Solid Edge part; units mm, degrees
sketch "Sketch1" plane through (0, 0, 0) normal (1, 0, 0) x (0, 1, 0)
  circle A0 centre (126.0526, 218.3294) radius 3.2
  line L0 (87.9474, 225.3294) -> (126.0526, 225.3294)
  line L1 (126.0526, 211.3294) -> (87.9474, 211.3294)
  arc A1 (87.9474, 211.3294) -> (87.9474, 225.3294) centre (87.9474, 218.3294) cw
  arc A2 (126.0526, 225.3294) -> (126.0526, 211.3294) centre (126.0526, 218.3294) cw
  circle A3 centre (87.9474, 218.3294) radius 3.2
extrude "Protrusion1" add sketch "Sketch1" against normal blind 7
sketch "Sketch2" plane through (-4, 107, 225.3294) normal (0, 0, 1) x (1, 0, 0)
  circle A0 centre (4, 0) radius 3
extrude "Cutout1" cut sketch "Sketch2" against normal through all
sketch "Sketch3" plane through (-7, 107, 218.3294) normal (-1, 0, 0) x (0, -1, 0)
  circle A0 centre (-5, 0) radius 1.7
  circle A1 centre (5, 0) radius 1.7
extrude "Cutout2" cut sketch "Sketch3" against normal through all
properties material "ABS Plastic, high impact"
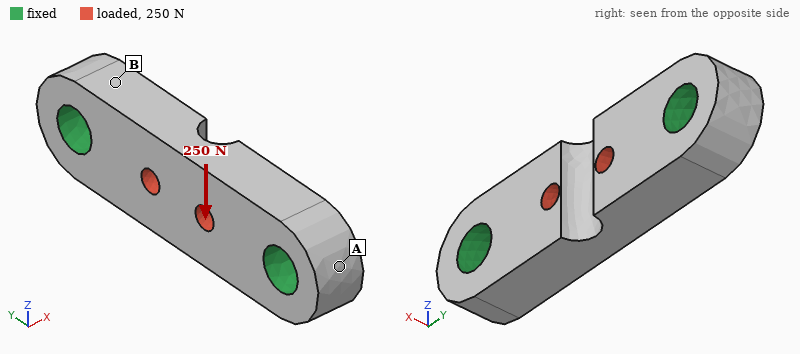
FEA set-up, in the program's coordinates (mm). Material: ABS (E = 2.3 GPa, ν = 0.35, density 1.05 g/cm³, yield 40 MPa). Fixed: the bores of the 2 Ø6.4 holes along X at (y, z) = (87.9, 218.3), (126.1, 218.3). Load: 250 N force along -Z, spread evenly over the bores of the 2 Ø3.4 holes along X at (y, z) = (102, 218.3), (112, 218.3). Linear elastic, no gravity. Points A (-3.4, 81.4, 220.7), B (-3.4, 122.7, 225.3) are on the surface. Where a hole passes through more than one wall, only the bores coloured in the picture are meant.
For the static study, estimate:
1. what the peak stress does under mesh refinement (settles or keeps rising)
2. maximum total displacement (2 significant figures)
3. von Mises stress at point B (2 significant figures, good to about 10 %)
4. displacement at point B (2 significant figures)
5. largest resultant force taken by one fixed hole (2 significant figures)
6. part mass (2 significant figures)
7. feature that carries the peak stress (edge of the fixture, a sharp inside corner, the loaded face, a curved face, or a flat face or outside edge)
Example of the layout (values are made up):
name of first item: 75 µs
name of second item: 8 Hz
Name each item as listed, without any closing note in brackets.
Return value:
what the peak stress does under mesh refinement: keeps rising
maximum total displacement: 51 µm
von Mises stress at point B: 2.8 MPa
displacement at point B: 12 µm
largest resultant force taken by one fixed hole: 130 N
part mass: 4.2 g
feature that carries the peak stress: a sharp inside corner
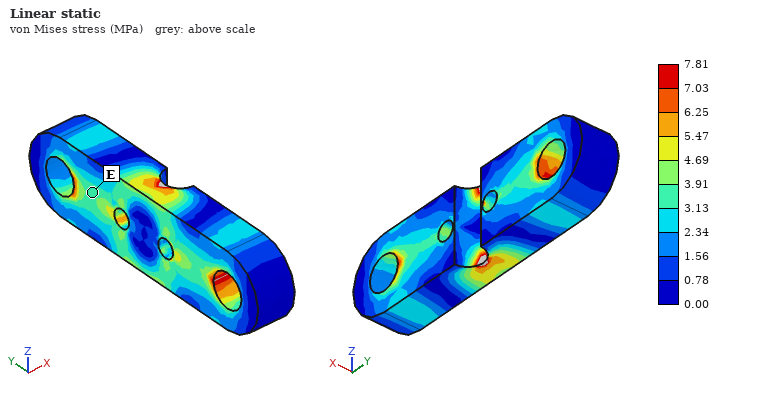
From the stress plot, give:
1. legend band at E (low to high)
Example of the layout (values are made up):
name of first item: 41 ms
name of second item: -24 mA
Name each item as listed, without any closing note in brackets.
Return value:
legend band at E: 3.13 to 3.91 MPa
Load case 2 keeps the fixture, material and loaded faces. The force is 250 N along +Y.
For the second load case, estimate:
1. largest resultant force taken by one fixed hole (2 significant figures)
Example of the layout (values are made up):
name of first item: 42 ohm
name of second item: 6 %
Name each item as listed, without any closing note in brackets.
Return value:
largest resultant force taken by one fixed hole: 130 N
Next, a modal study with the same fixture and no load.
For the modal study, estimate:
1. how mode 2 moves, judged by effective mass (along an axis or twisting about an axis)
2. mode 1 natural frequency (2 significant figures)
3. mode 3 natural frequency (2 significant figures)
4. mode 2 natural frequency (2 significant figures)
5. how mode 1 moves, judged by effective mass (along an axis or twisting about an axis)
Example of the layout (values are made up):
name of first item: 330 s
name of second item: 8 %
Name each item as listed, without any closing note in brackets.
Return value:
how mode 2 moves, judged by effective mass: along Z
mode 1 natural frequency: 7100 Hz
mode 3 natural frequency: 11 kHz
mode 2 natural frequency: 9000 Hz
how mode 1 moves, judged by effective mass: along X
